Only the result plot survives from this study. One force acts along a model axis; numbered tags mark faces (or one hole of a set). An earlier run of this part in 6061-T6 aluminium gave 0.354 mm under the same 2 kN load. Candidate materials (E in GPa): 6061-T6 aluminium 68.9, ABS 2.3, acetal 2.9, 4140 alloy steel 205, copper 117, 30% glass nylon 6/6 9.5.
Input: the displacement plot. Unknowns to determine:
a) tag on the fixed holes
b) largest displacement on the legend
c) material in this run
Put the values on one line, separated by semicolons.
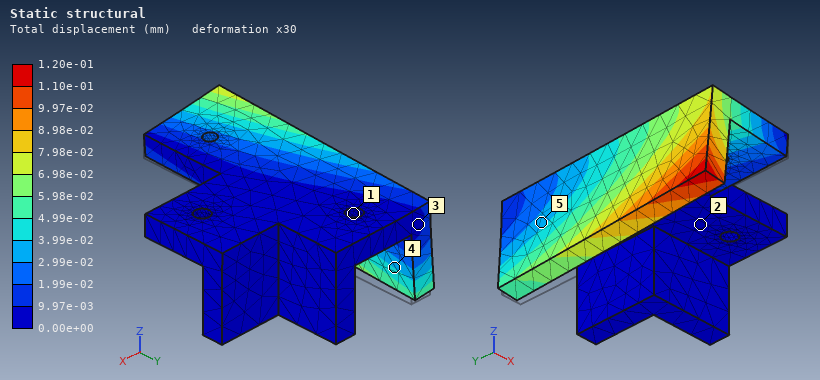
1; 1.20e-01 mm; 4140 alloy steel
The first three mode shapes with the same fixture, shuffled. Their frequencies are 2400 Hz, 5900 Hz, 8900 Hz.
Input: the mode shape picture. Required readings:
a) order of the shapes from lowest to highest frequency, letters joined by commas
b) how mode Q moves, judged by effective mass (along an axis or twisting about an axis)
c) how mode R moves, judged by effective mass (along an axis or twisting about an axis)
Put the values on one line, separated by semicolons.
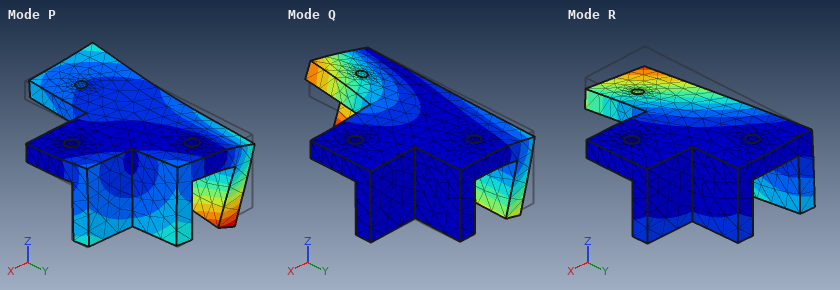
R, Q, P; along X; along Z
